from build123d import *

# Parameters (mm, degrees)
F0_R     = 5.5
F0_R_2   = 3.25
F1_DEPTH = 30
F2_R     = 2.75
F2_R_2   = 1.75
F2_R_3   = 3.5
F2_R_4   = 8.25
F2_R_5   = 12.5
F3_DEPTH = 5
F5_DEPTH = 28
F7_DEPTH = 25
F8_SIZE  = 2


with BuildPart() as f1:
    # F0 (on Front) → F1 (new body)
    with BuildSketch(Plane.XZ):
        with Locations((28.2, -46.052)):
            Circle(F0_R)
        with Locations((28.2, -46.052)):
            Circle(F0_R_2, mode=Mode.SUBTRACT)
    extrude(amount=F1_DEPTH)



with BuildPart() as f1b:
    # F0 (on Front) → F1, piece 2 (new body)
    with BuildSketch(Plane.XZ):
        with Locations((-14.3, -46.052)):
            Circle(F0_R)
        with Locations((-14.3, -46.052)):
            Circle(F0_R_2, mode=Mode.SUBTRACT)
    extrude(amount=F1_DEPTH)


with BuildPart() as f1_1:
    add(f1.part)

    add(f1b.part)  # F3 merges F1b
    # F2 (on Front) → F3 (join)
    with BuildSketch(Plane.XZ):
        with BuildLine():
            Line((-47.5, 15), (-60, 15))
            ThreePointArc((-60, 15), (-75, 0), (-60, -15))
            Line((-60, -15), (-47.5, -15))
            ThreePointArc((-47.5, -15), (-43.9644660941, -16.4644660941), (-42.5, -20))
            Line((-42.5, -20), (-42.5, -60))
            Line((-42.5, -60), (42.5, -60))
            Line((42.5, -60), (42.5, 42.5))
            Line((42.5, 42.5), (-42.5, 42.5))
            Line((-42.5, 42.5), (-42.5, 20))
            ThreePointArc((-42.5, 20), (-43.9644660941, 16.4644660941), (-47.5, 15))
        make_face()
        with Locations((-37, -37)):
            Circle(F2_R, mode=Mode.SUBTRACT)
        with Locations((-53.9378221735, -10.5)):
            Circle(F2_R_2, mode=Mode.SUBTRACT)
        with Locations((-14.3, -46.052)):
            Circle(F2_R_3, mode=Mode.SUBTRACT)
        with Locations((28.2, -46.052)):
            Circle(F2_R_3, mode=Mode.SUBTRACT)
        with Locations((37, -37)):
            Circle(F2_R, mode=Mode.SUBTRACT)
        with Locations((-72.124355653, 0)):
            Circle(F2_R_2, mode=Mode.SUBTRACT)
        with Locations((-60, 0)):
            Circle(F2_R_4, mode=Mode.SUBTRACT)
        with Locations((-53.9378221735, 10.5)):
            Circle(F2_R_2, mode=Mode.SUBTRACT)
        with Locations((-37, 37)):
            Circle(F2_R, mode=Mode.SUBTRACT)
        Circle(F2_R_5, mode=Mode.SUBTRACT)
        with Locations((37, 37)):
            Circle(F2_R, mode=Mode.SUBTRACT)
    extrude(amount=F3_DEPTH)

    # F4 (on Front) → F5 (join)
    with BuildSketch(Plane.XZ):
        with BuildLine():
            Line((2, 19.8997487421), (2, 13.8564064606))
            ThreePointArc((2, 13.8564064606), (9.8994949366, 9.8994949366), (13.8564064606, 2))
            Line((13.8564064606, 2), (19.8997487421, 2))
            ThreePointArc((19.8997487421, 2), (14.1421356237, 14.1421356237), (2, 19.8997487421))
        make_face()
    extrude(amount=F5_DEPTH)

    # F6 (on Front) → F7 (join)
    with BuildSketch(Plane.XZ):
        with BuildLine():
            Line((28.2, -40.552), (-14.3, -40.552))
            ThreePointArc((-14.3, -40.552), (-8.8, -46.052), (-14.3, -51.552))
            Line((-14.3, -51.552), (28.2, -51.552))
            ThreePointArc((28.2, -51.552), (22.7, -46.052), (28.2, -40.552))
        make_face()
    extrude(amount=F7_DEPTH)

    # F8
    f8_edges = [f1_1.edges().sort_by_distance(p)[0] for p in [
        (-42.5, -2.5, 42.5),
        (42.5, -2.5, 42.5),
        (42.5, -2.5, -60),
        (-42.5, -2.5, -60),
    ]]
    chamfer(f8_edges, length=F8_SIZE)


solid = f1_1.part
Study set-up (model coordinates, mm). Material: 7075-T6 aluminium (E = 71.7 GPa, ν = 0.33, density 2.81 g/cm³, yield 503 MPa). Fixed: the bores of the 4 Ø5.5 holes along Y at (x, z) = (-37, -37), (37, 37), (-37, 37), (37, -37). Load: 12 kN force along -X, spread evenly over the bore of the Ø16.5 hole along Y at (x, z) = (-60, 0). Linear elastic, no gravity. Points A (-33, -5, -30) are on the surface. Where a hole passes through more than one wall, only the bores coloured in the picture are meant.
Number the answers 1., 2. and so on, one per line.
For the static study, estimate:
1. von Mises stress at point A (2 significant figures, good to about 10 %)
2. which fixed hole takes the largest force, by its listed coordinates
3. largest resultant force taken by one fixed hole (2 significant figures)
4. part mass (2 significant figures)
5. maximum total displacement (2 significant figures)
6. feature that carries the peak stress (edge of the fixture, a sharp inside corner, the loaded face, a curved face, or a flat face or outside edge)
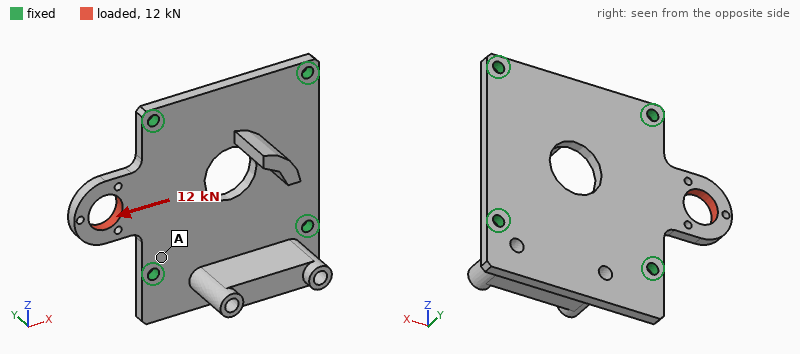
1. 52 MPa
2. (-37, -37)
3. 3.9 kN
4. 160 g
5. 0.13 mm
6. a curved face
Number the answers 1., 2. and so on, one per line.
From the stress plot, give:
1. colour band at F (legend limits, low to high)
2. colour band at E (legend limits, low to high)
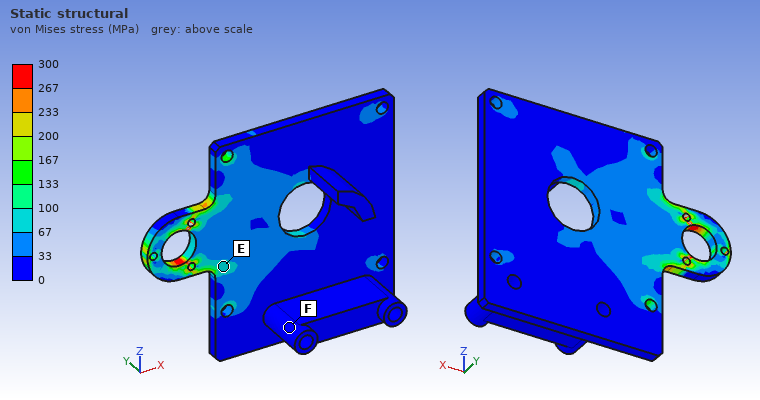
1. 0 to 33 MPa
2. 67 to 100 MPa
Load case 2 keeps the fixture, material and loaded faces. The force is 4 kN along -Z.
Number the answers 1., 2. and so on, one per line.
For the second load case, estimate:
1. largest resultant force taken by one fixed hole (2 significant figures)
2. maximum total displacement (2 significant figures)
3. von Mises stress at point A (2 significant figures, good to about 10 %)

1. 2.2 kN
2. 0.15 mm
3. 27 MPa
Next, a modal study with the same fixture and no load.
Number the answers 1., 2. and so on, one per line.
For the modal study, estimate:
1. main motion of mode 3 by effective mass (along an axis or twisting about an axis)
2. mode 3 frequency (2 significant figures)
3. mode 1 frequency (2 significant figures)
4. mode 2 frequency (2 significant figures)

1. along Y
2. 3400 Hz
3. 2200 Hz
4. 2700 Hz
